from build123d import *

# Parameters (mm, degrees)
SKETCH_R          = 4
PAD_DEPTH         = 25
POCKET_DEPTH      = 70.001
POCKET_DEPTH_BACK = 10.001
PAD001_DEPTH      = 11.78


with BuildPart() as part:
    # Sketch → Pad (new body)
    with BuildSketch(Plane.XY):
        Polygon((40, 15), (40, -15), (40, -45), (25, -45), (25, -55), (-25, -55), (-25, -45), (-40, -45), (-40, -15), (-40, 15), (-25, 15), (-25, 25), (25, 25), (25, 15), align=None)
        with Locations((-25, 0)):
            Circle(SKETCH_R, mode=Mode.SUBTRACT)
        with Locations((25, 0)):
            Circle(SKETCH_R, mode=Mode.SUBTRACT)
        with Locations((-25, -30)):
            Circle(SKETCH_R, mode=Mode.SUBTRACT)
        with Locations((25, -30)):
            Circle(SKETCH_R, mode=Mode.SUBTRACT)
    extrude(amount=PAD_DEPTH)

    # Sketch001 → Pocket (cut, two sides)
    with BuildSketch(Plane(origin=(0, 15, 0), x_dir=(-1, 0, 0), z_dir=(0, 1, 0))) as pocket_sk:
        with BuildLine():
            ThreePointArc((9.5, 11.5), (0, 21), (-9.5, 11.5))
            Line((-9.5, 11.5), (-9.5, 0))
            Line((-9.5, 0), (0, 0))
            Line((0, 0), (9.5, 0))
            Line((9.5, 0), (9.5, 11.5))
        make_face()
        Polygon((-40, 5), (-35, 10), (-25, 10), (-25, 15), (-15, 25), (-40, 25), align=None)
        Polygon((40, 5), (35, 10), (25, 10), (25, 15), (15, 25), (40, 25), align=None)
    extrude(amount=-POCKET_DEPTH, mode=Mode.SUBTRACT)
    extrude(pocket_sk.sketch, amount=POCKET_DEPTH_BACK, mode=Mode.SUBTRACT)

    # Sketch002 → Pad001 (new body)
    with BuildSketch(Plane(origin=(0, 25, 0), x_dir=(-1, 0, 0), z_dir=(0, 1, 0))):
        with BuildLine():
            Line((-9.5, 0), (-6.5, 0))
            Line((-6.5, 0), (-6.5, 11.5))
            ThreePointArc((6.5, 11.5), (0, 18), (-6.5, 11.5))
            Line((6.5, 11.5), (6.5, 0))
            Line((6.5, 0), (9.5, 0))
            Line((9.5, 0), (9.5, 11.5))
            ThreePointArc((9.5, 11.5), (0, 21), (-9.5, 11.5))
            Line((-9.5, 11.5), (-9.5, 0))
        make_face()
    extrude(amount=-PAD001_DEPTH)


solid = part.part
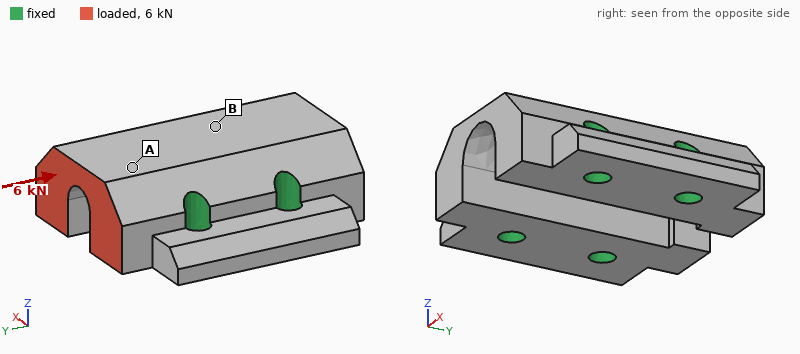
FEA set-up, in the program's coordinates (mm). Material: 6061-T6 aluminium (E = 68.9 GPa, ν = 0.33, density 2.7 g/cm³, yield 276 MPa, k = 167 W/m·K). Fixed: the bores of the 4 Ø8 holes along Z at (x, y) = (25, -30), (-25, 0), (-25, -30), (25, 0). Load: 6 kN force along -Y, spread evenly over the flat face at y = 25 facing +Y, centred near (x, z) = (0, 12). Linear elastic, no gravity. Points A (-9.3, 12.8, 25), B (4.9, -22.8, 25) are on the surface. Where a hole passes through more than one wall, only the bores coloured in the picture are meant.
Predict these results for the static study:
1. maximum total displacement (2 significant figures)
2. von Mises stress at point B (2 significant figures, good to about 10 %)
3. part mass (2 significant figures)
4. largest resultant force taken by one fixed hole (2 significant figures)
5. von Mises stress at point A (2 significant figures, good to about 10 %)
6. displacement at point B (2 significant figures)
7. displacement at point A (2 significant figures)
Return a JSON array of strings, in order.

["6.7 µm", "2.4 MPa", "210 g", "2.3 kN", "6.1 MPa", "1.3 µm", "4.3 µm"]
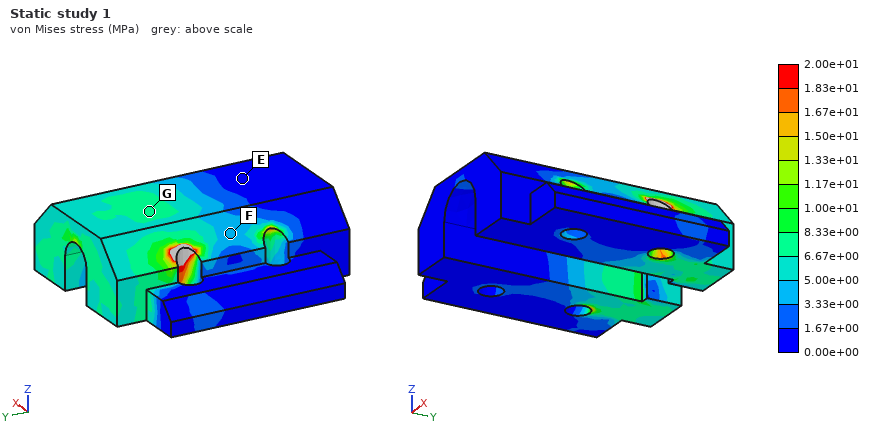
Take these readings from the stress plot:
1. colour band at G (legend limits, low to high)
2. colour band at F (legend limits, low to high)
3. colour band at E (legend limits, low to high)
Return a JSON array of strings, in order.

["6.67e+00 to 8.33e+00 MPa", "3.33e+00 to 5.00e+00 MPa", "0.00e+00 to 1.67e+00 MPa"]
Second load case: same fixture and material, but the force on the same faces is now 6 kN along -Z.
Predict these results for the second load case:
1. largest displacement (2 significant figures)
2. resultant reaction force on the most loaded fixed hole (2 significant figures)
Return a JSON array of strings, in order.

["31 µm", "4.0 kN"]
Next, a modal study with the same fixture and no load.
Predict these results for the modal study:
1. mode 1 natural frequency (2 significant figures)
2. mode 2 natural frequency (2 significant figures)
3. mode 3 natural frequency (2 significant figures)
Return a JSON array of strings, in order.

["15 kHz", "17 kHz", "17 kHz"]
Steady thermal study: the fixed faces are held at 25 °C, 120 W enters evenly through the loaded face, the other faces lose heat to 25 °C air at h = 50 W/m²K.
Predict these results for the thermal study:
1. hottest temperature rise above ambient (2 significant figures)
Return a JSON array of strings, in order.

["23 K"]
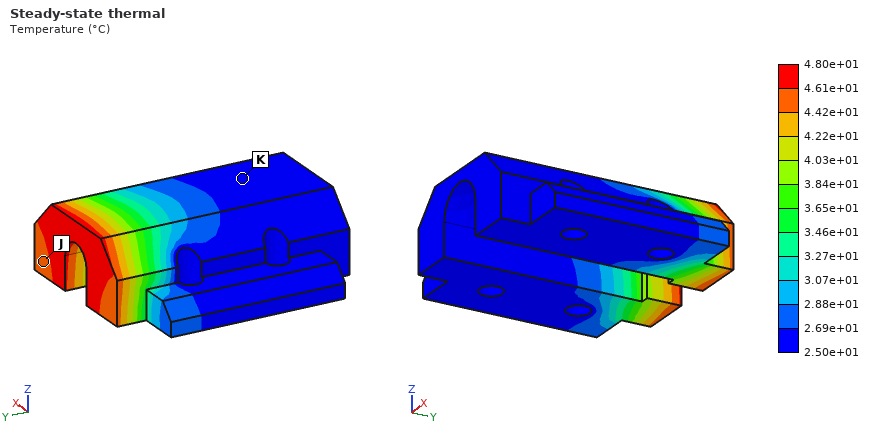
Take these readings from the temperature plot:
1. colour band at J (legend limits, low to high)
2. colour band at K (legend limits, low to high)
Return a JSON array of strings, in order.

["4.42e+01 to 4.61e+01 °C", "2.50e+01 to 2.69e+01 °C"]
